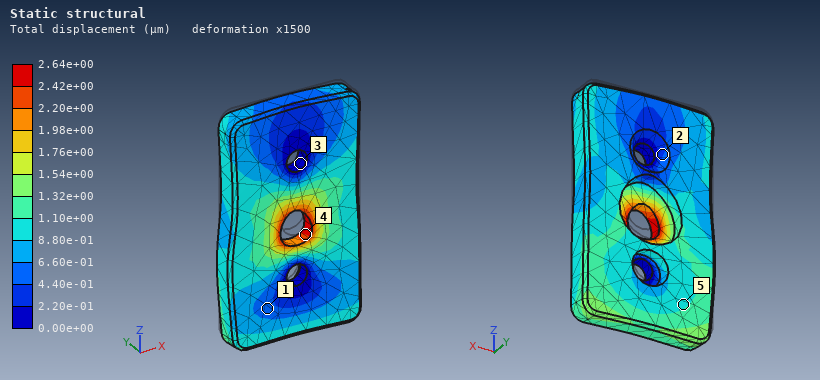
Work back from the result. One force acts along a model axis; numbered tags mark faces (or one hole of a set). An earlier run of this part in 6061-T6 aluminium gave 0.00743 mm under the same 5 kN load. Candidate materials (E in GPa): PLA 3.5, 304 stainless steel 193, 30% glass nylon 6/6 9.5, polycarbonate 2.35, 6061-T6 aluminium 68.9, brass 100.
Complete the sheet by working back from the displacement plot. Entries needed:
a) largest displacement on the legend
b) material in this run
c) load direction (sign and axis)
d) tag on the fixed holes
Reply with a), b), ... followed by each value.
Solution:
a) 2.64e+00 µm
b) 304 stainless steel
c) -Z
d) 3
